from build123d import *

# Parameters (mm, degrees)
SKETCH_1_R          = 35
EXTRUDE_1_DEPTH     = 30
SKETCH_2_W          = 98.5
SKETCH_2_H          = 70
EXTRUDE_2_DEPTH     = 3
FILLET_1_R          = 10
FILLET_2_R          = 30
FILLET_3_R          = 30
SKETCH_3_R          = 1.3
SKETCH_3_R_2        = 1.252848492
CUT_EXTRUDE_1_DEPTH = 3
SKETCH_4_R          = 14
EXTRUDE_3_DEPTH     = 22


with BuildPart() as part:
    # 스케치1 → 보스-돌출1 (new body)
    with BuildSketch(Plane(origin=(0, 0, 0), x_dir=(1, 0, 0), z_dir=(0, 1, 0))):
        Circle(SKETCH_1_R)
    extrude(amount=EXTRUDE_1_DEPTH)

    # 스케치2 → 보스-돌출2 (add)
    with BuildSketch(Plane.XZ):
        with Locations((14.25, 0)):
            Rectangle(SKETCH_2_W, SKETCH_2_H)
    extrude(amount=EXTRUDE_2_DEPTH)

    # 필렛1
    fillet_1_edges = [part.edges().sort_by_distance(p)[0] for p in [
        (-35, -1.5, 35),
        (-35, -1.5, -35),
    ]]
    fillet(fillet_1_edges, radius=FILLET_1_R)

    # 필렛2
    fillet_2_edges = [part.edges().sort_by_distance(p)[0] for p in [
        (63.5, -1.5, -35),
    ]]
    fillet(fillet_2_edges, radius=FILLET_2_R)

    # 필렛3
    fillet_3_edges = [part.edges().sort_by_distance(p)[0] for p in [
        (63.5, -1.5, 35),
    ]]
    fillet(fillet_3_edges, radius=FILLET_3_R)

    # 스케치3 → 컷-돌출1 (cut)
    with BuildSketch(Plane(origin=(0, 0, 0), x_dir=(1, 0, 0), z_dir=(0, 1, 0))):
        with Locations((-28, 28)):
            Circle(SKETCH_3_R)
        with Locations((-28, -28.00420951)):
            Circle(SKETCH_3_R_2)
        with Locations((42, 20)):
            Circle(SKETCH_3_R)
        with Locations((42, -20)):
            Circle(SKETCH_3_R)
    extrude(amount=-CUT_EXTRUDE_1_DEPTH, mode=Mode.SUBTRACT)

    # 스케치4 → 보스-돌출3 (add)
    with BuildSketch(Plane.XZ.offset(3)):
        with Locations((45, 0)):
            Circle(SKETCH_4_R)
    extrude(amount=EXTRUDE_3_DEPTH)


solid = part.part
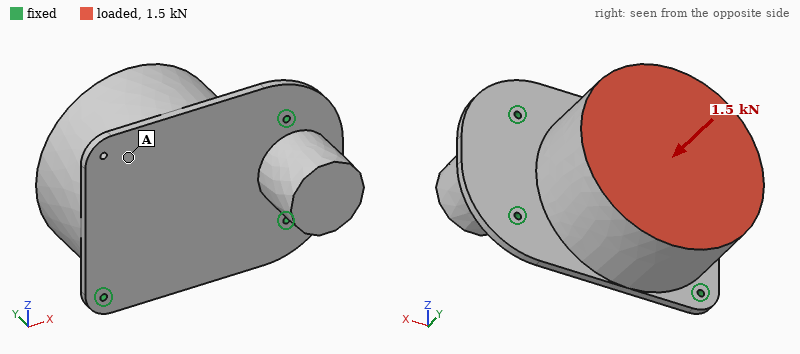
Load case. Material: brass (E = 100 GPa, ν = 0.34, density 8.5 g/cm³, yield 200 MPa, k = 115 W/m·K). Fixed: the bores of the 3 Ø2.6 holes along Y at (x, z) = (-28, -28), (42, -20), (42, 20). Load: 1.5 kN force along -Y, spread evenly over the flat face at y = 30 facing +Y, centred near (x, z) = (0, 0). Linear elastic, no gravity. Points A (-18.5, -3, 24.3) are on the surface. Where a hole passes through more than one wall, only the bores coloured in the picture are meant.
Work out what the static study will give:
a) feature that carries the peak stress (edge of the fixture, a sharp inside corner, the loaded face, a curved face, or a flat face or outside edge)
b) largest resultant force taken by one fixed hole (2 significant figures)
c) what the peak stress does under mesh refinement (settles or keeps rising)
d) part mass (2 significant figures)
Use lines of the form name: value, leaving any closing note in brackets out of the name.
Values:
feature that carries the peak stress: edge of the fixture
largest resultant force taken by one fixed hole: 950 N
what the peak stress does under mesh refinement: keeps rising
part mass: 1.3 kg
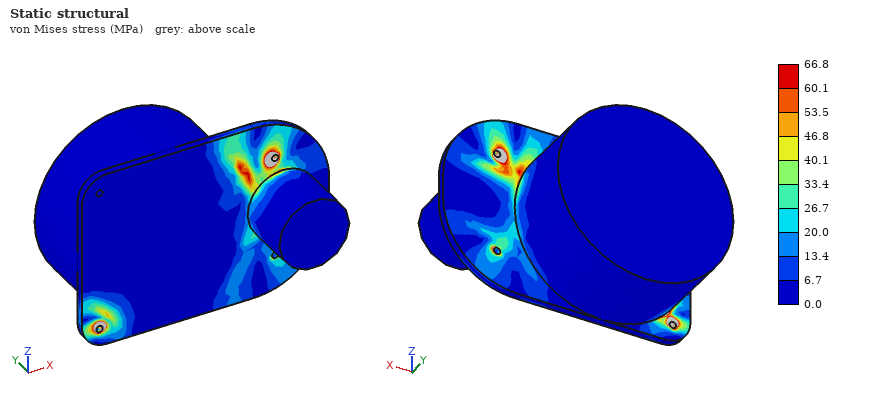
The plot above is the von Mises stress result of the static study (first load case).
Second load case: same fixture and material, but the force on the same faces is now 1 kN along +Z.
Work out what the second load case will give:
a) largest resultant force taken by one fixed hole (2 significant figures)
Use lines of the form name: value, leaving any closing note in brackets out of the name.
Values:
largest resultant force taken by one fixed hole: 900 N
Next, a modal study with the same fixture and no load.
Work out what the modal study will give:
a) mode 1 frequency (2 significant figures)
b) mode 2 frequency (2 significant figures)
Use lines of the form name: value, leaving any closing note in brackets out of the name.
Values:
mode 1 frequency: 730 Hz
mode 2 frequency: 1800 Hz
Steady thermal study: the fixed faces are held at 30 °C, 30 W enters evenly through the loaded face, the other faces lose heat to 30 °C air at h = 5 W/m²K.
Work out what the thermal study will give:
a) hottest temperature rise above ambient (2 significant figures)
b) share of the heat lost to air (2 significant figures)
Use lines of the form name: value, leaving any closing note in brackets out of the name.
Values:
hottest temperature rise above ambient: 20 K
share of the heat lost to air: 4.4 %
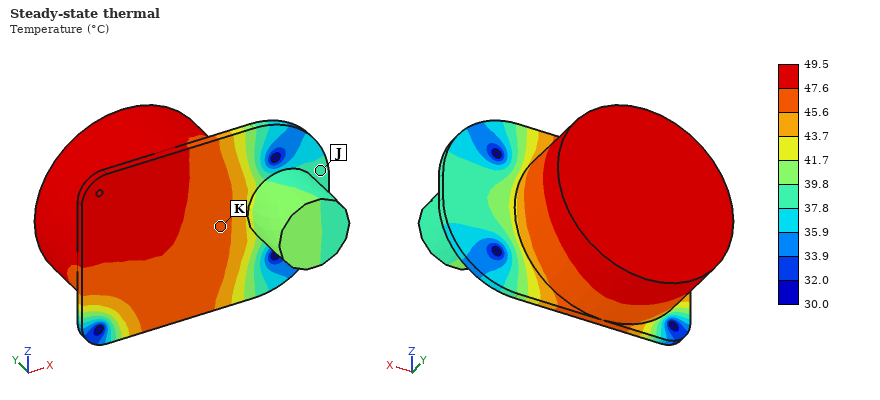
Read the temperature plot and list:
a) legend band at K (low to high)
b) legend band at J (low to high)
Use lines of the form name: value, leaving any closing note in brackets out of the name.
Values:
legend band at K: 45.6 to 47.6 °C
legend band at J: 37.8 to 39.8 °C
